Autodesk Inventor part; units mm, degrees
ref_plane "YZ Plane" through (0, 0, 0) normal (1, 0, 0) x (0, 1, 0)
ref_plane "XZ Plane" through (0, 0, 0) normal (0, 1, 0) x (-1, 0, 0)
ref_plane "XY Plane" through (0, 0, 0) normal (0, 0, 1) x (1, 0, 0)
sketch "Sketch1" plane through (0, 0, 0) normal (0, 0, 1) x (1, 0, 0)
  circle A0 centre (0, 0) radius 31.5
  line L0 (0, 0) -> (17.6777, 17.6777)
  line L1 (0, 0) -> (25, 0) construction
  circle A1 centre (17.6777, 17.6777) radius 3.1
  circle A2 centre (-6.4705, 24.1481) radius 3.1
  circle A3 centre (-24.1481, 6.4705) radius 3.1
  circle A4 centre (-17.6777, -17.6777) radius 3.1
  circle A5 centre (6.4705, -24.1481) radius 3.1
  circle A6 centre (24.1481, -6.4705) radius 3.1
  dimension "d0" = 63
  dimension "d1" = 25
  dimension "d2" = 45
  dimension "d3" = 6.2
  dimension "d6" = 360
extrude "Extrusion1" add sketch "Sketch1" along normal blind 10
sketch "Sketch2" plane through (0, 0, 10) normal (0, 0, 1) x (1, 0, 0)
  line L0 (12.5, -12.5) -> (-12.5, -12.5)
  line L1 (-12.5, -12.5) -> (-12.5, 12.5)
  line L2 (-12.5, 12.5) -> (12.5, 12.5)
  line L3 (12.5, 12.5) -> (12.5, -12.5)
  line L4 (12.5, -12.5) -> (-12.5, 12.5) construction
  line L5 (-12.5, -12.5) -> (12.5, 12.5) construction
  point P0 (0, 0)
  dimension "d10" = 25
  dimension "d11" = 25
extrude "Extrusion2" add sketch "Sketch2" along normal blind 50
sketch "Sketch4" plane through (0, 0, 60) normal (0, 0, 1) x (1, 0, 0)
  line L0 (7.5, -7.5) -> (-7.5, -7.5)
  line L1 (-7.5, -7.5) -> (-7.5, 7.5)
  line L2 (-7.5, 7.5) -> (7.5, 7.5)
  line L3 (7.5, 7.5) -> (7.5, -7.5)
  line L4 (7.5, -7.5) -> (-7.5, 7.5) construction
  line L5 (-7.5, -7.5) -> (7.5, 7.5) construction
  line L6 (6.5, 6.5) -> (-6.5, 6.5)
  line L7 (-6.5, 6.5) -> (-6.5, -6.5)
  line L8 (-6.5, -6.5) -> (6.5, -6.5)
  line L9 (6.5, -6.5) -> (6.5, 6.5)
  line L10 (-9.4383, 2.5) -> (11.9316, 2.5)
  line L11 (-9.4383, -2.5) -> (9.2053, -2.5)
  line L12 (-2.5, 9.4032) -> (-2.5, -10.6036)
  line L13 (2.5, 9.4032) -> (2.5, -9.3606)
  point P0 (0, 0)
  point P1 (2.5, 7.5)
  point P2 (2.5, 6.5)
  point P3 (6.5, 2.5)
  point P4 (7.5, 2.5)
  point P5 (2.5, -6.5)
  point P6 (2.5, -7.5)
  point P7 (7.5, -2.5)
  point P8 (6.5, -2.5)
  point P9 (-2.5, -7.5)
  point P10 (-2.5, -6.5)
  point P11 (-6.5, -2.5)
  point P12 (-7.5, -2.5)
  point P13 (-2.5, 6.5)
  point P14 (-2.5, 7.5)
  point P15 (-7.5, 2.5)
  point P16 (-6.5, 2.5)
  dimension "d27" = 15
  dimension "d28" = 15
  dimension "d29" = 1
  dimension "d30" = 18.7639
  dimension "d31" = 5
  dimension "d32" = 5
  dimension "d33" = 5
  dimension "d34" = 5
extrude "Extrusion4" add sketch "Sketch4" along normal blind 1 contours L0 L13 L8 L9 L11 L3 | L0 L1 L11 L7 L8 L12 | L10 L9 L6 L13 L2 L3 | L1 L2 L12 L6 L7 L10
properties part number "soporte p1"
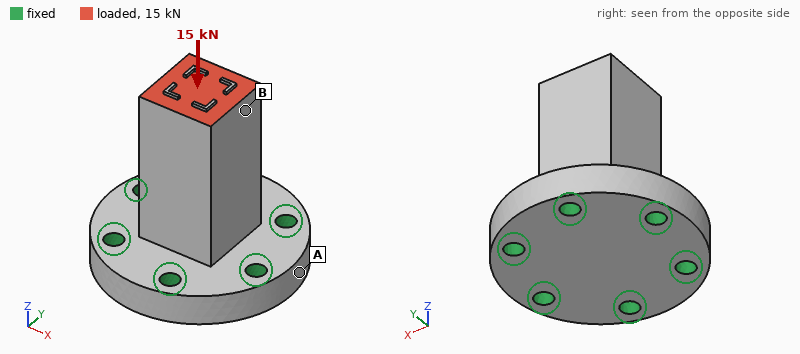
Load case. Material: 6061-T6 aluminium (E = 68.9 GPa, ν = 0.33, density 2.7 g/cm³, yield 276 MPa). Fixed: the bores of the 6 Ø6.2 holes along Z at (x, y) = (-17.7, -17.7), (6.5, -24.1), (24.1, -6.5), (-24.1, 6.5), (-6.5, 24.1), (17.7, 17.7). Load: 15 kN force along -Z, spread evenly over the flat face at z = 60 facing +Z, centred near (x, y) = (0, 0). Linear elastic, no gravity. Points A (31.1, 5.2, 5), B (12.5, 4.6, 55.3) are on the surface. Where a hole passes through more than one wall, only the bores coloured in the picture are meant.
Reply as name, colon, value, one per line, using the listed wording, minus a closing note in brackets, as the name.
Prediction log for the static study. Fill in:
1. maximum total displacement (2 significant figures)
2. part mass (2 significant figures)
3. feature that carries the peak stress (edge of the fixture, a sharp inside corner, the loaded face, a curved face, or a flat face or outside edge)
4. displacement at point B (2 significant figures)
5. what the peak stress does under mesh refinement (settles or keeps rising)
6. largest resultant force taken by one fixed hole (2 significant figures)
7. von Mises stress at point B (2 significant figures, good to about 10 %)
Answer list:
maximum total displacement: 31 µm
part mass: 160 g
feature that carries the peak stress: edge of the fixture
displacement at point B: 29 µm
what the peak stress does under mesh refinement: keeps rising
largest resultant force taken by one fixed hole: 2.8 kN
von Mises stress at point B: 25 MPa
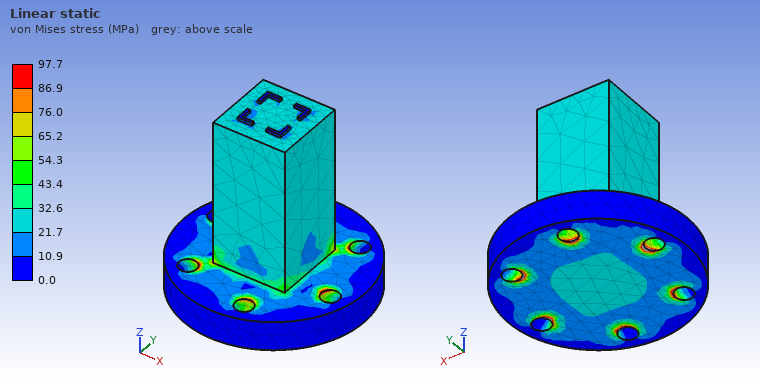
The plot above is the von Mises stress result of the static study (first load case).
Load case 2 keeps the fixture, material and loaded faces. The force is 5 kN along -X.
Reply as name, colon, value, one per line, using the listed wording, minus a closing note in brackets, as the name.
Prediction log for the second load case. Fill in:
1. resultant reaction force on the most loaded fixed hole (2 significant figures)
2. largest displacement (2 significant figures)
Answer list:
resultant reaction force on the most loaded fixed hole: 4.1 kN
largest displacement: 0.18 mm
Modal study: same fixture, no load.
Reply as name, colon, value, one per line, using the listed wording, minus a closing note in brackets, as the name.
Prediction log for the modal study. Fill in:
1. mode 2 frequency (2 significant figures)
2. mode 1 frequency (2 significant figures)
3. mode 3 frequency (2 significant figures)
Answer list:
mode 2 frequency: 5200 Hz
mode 1 frequency: 5200 Hz
mode 3 frequency: 13 kHz
